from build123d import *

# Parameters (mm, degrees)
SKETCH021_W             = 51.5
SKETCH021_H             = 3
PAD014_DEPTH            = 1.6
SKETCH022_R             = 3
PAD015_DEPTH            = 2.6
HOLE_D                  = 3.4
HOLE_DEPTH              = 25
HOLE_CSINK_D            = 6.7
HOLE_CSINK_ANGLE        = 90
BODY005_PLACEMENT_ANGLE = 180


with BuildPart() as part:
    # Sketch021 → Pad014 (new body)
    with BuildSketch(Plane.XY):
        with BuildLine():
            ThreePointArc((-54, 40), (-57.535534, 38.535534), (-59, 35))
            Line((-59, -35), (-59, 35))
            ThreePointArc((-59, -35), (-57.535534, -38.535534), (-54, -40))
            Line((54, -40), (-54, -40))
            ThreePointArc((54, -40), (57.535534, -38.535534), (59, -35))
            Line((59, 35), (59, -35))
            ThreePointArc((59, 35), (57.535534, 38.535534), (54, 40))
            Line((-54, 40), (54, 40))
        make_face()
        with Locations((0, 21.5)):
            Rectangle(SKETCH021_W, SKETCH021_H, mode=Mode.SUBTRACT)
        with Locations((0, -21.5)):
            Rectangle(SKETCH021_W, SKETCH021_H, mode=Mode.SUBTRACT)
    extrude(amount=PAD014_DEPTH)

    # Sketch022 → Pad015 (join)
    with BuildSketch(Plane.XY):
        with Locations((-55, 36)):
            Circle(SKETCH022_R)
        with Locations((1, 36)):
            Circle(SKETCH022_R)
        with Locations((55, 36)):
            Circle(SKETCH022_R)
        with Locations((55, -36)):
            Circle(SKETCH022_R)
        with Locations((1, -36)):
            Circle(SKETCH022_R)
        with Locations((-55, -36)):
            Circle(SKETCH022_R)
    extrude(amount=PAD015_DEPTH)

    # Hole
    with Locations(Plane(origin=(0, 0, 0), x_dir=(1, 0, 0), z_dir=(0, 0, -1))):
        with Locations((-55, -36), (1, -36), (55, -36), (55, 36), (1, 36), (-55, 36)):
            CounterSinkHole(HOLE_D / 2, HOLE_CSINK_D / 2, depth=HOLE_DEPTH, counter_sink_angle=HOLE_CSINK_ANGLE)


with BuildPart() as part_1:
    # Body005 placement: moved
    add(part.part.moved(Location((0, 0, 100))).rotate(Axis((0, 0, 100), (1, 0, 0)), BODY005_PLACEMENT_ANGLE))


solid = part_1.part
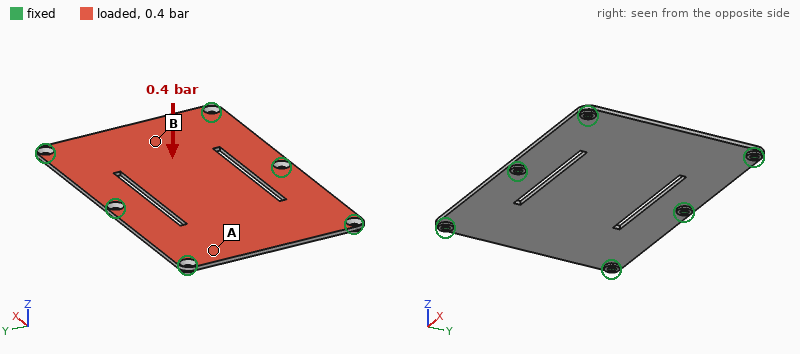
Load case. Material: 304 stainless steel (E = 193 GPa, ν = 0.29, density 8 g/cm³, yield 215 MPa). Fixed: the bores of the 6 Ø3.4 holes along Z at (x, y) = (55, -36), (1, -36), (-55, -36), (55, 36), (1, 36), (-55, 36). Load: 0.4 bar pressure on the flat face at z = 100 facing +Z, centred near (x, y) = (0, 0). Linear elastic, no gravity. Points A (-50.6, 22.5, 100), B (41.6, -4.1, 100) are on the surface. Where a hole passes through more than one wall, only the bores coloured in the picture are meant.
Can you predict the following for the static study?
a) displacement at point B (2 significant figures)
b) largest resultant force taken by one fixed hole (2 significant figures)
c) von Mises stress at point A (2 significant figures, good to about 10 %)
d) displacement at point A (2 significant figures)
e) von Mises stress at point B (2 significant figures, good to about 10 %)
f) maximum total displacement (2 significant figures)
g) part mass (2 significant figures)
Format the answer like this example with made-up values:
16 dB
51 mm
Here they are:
0.088 mm
160 N
11 MPa
0.035 mm
28 MPa
0.16 mm
120 g
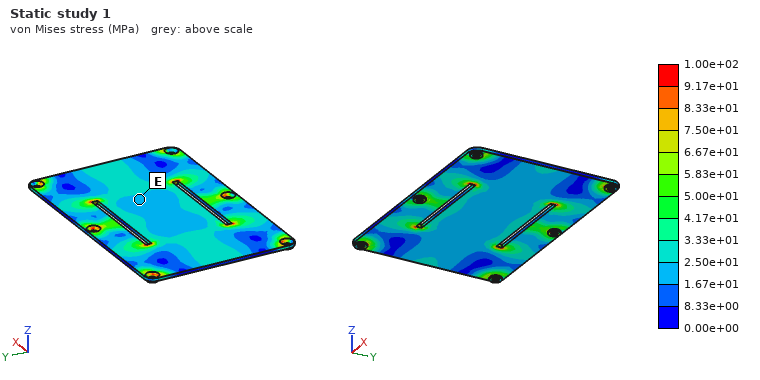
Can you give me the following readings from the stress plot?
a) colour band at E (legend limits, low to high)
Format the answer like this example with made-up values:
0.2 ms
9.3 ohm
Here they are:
1.67e+01 to 2.50e+01 MPa
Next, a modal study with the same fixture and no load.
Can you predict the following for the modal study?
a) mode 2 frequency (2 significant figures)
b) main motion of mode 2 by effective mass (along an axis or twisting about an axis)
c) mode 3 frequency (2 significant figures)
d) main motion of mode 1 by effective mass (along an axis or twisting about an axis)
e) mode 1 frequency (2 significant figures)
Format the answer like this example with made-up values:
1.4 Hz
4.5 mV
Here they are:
1300 Hz
twisting about Y
1800 Hz
along Z
860 Hz
